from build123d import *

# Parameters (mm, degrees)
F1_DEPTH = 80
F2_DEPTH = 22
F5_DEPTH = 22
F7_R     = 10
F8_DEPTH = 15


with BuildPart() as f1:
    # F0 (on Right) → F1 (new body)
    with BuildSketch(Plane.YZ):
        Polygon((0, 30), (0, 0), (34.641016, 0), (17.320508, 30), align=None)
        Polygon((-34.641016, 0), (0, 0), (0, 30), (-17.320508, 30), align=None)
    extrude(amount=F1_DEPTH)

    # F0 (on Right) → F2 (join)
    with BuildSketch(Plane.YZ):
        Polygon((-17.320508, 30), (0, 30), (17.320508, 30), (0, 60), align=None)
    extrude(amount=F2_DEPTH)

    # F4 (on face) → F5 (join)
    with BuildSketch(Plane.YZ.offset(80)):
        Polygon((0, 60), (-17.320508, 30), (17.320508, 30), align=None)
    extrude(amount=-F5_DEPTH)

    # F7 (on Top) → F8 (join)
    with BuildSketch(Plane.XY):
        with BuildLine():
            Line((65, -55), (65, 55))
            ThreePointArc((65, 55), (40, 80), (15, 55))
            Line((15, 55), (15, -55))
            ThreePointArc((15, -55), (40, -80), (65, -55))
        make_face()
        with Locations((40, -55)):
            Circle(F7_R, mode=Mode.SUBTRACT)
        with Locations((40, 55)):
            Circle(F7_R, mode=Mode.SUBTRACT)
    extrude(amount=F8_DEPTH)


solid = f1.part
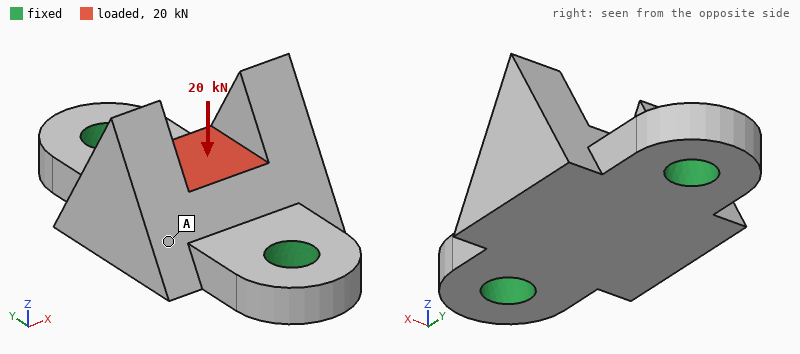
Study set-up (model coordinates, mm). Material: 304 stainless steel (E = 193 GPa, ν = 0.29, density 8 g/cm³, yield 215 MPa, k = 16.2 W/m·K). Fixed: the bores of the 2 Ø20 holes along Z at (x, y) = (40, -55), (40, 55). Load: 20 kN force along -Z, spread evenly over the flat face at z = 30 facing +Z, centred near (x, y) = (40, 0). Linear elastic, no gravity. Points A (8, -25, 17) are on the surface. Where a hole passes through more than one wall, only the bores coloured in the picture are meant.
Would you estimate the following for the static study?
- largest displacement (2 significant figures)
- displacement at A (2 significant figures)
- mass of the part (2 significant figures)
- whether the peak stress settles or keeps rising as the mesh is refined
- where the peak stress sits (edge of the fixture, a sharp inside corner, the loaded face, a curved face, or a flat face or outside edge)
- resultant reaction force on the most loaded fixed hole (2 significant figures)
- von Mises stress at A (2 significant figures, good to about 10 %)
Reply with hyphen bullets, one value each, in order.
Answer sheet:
- 18 µm
- 15 µm
- 1.6 kg
- keeps rising
- edge of the fixture
- 11 kN
- 15 MPa
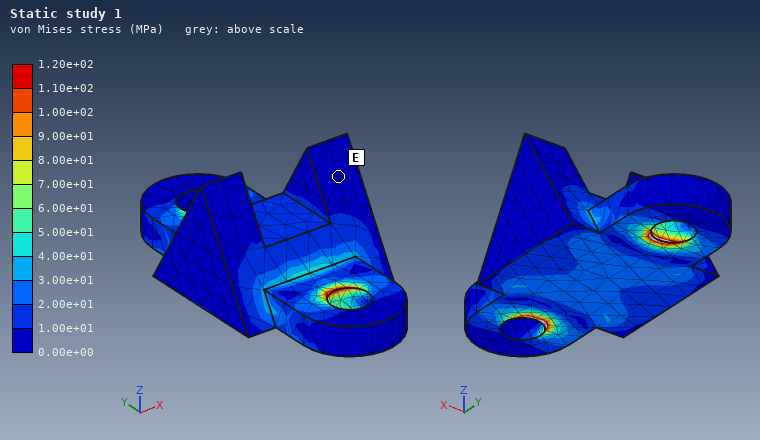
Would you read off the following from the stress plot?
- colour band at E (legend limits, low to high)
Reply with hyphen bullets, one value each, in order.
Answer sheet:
- 0.00e+00 to 1.00e+01 MPa
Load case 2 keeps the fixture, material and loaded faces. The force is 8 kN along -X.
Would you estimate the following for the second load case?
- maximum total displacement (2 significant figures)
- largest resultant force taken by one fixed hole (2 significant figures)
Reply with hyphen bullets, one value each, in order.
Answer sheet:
- 37 µm
- 4.0 kN
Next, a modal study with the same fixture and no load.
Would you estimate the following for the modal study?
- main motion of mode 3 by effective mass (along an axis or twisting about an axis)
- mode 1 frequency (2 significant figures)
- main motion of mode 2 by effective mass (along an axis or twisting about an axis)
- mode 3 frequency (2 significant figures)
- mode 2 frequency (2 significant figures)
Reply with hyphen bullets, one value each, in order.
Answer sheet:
- along X
- 2900 Hz
- along Z
- 8300 Hz
- 4900 Hz
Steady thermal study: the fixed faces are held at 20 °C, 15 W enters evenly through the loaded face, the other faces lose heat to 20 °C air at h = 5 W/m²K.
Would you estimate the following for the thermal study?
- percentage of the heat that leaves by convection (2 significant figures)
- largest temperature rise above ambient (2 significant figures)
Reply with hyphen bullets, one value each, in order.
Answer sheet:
- 11 %
- 28 K
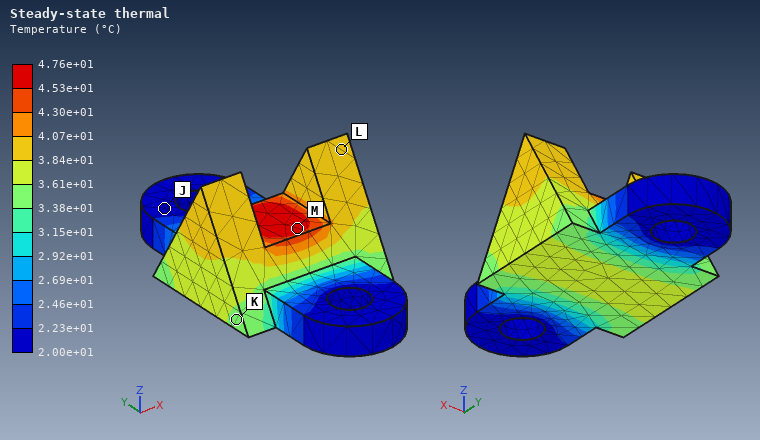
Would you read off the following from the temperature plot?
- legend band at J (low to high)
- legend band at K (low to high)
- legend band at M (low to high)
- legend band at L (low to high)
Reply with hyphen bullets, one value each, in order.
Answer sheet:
- 2.00e+01 to 2.23e+01 °C
- 3.38e+01 to 3.61e+01 °C
- 4.53e+01 to 4.76e+01 °C
- 3.84e+01 to 4.07e+01 °C
